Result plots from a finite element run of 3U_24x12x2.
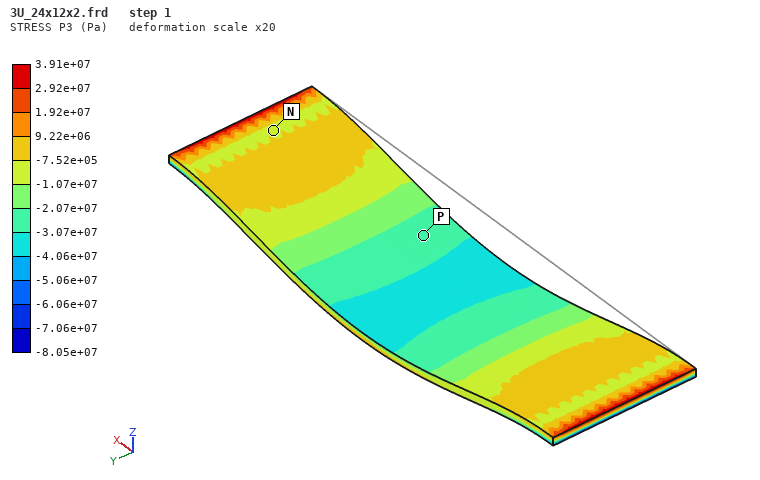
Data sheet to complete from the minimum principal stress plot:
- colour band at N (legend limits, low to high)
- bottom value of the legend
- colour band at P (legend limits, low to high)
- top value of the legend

-1.07e+07 to -7.52e+05 Pa
-8.05e+07 Pa
-3.07e+07 to -2.07e+07 Pa
3.91e+07 Pa
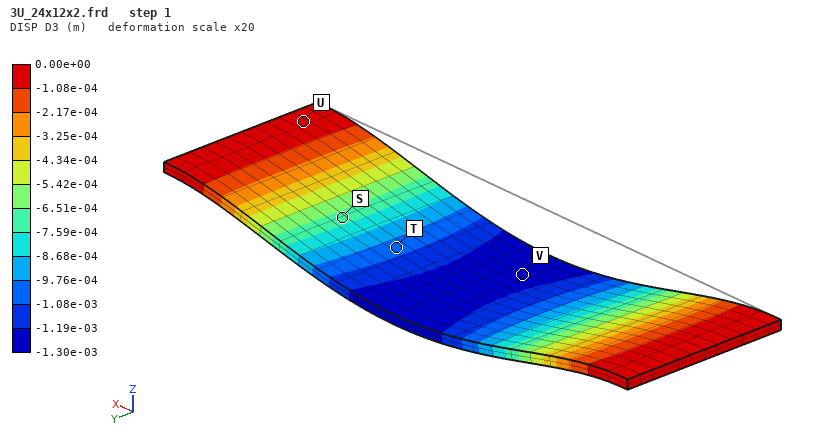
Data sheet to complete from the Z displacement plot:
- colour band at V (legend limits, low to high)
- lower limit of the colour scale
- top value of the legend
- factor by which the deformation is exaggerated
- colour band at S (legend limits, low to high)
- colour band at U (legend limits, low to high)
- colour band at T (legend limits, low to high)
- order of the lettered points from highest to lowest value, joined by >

-1.30e-03 to -1.19e-03 m
-1.30e-03 m
0.00e+00 m
20
-7.59e-04 to -6.51e-04 m
-1.08e-04 to 0.00e+00 m
-1.08e-03 to -9.76e-04 m
U > S > T > V
